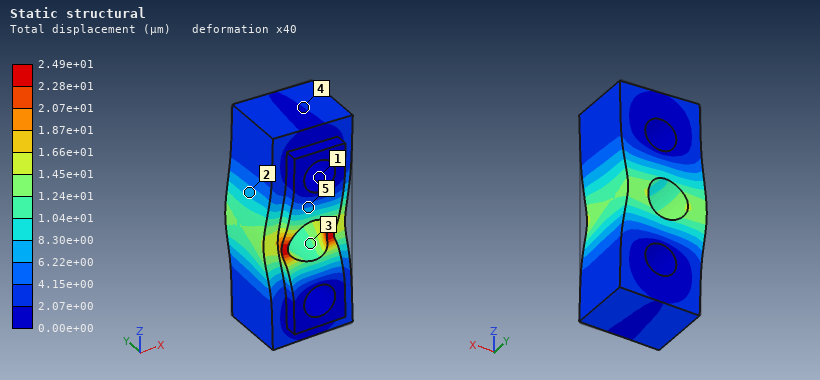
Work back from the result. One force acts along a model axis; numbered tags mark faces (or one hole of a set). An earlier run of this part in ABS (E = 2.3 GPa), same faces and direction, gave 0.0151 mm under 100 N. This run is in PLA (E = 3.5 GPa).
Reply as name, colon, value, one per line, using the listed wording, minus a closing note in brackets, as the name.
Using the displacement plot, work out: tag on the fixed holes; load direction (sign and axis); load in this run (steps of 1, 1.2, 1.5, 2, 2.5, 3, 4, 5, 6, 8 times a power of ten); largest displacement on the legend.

tag on the fixed holes: 1
load direction: -X
load in this run: 250 N
largest displacement on the legend: 2.49e+01 µm
